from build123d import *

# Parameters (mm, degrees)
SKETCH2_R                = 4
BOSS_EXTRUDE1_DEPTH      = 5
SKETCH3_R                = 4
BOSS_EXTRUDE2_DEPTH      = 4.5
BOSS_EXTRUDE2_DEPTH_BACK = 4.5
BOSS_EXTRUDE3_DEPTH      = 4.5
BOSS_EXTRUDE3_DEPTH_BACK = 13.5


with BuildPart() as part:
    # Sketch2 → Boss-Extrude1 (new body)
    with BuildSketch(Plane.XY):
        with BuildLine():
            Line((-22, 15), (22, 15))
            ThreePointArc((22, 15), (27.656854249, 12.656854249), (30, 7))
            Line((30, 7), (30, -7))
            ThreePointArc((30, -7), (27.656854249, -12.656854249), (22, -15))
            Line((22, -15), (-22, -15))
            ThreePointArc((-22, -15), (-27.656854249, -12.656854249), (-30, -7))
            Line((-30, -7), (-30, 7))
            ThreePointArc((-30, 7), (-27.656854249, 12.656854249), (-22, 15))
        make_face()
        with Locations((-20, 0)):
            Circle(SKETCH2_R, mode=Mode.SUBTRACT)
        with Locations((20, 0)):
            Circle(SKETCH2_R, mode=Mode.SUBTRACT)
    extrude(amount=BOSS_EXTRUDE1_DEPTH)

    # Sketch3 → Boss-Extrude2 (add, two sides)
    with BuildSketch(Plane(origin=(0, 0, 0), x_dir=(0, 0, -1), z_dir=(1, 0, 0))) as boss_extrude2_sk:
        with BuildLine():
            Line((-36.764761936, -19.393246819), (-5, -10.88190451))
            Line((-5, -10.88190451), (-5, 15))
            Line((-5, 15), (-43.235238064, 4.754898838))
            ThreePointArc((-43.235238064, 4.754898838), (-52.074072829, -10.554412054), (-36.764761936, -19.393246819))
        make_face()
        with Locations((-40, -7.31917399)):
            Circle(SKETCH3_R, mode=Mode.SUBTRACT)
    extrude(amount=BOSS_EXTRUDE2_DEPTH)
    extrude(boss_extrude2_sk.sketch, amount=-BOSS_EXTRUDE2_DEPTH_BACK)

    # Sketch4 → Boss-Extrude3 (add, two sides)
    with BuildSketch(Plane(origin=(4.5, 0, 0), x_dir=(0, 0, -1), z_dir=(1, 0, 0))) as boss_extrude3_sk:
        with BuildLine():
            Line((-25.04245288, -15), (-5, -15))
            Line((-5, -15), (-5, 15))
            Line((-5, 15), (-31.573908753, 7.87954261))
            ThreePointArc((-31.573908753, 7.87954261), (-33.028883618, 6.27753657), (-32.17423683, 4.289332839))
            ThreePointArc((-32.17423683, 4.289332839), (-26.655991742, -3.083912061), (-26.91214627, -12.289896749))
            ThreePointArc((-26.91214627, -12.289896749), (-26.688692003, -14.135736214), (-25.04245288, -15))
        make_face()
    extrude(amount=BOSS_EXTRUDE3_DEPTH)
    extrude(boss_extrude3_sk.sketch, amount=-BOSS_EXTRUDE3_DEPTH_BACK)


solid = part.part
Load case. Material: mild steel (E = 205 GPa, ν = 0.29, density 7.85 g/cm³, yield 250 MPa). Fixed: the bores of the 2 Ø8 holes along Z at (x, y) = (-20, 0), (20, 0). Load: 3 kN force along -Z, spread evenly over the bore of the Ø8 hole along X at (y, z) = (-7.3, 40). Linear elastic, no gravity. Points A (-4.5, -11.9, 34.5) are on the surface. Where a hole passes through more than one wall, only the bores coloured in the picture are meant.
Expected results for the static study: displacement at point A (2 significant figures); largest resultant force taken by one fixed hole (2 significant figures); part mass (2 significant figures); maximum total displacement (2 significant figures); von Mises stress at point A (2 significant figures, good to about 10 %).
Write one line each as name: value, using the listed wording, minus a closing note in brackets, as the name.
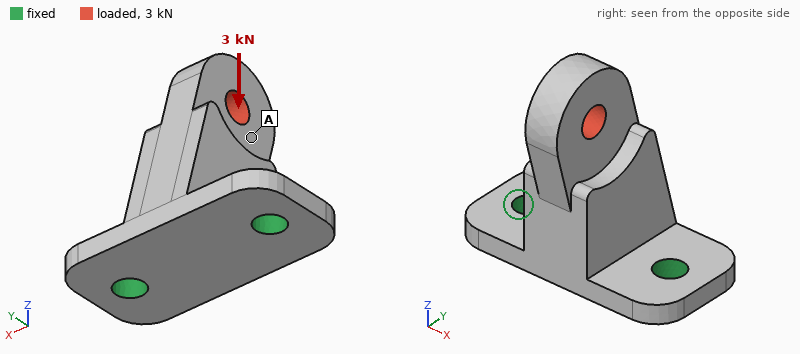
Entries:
displacement at point A: 33 µm
largest resultant force taken by one fixed hole: 1.6 kN
part mass: 190 g
maximum total displacement: 47 µm
von Mises stress at point A: 24 MPa
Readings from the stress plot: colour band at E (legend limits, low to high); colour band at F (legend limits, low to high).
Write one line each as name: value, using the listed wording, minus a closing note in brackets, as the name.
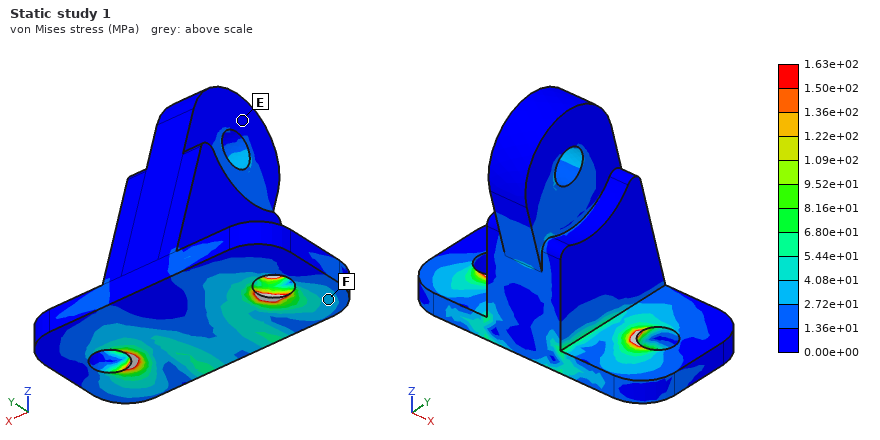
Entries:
colour band at E: 0.00e+00 to 1.36e+01 MPa
colour band at F: 2.72e+01 to 4.08e+01 MPa
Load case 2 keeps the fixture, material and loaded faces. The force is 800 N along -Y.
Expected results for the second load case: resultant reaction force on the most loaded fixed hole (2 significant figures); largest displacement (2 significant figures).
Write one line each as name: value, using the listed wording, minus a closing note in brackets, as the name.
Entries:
resultant reaction force on the most loaded fixed hole: 400 N
largest displacement: 63 µm
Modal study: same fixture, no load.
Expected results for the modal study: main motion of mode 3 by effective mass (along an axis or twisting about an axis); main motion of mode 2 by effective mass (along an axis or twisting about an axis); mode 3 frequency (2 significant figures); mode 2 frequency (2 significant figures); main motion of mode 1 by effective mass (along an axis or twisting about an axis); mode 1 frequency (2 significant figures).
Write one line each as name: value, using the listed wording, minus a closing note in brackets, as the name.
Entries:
main motion of mode 3 by effective mass: along Z
main motion of mode 2 by effective mass: along X
mode 3 frequency: 9100 Hz
mode 2 frequency: 4800 Hz
main motion of mode 1 by effective mass: along Y
mode 1 frequency: 2800 Hz
